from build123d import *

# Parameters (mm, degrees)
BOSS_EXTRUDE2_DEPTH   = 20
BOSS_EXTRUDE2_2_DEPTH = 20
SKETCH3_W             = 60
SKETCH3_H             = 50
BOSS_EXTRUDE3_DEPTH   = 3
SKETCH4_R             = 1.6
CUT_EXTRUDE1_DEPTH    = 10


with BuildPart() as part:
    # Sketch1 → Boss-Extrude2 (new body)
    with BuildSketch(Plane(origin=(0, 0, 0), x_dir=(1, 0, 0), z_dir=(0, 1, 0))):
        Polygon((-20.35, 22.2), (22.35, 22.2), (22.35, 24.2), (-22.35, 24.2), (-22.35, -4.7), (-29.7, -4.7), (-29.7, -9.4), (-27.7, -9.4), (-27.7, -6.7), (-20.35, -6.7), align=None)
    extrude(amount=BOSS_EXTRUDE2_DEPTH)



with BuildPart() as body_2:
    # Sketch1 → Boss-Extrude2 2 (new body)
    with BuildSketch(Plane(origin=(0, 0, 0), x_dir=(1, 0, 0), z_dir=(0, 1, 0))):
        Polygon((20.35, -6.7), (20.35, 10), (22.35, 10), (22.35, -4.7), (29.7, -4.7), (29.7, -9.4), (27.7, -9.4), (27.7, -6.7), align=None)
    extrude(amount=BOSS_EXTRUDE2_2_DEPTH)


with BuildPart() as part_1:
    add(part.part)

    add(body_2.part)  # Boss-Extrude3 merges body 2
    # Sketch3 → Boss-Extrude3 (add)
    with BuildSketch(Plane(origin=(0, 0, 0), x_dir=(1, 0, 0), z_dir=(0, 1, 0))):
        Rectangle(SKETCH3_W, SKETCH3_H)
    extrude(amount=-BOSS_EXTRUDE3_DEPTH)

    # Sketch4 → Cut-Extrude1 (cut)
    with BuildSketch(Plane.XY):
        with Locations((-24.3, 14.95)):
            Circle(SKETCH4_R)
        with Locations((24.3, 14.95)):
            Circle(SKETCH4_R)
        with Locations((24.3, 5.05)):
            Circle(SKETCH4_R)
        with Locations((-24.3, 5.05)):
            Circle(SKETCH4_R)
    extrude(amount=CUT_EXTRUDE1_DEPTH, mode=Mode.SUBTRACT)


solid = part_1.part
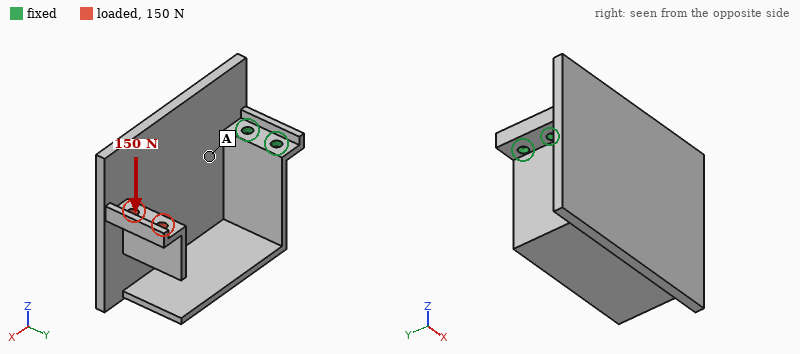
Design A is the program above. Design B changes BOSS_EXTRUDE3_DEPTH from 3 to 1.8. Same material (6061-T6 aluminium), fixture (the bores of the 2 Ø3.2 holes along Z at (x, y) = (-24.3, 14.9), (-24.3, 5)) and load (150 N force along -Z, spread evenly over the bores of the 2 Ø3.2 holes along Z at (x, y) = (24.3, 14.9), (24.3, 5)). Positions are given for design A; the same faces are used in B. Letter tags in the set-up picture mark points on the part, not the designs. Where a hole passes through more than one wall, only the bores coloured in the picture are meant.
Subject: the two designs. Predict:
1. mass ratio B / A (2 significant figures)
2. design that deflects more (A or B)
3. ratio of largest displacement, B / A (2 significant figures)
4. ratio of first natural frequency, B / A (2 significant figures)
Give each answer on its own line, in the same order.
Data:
0.73
B
1.4
0.85
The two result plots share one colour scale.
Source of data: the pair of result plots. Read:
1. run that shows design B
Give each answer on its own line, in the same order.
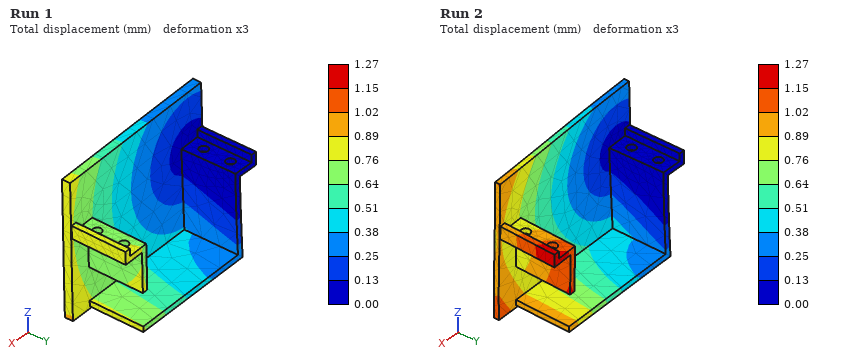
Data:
Run 2
